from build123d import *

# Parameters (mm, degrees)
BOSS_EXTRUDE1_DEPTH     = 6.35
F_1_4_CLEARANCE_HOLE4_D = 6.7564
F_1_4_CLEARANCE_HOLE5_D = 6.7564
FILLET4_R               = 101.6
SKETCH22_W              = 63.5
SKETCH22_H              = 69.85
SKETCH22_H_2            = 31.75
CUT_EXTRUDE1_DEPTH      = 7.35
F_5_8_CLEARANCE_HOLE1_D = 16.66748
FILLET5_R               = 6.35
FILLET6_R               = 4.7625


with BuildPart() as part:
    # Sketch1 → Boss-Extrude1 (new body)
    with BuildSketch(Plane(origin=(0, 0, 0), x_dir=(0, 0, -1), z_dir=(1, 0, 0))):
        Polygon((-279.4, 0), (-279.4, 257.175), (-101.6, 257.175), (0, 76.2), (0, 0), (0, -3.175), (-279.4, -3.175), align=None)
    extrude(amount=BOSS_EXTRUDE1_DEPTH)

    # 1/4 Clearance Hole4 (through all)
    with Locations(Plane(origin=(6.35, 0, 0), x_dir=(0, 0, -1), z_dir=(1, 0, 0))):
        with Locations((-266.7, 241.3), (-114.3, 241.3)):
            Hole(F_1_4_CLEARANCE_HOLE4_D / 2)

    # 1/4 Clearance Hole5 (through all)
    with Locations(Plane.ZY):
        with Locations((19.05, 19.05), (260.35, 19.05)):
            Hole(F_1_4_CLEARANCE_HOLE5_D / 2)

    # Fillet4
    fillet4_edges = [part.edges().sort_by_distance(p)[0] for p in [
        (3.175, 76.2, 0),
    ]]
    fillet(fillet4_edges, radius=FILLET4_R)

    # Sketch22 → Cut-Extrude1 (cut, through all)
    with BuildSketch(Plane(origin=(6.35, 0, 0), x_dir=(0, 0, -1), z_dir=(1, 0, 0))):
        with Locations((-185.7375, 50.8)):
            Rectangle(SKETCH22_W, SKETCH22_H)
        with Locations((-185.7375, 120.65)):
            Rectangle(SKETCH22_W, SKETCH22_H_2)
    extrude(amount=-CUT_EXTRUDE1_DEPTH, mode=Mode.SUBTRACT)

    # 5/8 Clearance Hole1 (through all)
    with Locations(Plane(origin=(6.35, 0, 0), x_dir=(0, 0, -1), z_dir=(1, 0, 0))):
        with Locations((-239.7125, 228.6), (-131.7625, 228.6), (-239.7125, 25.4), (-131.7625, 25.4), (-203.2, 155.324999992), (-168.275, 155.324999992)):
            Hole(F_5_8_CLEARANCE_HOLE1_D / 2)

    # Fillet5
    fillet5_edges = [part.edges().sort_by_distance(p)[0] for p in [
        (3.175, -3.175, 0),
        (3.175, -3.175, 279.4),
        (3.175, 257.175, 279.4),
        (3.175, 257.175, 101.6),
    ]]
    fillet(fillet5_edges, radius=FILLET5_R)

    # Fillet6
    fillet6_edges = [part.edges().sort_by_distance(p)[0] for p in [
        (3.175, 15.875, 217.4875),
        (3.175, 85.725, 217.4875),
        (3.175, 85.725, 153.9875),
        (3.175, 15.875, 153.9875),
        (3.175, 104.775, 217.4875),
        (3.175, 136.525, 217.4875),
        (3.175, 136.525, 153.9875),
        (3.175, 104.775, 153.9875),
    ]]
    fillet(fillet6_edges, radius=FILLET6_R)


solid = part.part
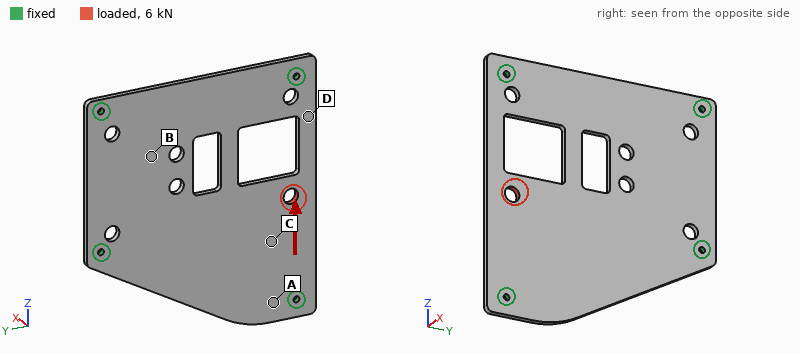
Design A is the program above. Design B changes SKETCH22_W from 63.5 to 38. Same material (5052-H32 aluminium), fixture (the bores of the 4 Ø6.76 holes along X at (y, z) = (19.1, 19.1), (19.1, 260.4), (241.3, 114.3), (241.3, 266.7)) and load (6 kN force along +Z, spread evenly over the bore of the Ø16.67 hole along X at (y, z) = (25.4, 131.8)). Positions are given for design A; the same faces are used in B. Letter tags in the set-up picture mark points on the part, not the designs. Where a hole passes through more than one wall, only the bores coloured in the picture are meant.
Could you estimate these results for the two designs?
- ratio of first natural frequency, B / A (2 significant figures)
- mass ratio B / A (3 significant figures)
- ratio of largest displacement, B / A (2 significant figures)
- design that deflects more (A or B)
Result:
0.99
1.05
0.86
A
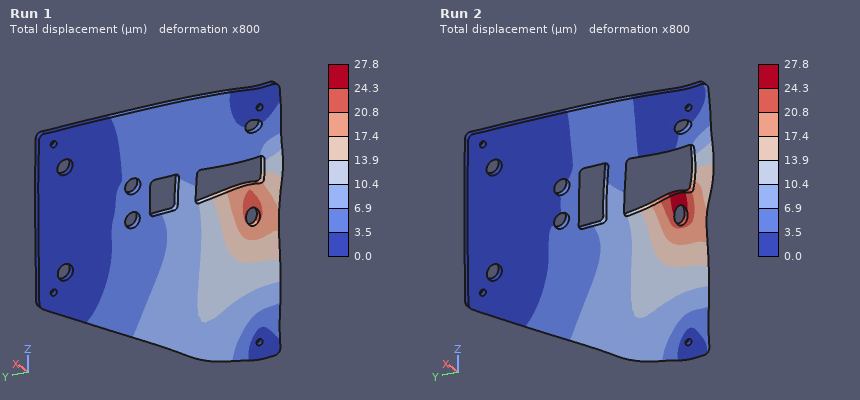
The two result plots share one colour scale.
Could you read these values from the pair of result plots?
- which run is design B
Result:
Run 1
